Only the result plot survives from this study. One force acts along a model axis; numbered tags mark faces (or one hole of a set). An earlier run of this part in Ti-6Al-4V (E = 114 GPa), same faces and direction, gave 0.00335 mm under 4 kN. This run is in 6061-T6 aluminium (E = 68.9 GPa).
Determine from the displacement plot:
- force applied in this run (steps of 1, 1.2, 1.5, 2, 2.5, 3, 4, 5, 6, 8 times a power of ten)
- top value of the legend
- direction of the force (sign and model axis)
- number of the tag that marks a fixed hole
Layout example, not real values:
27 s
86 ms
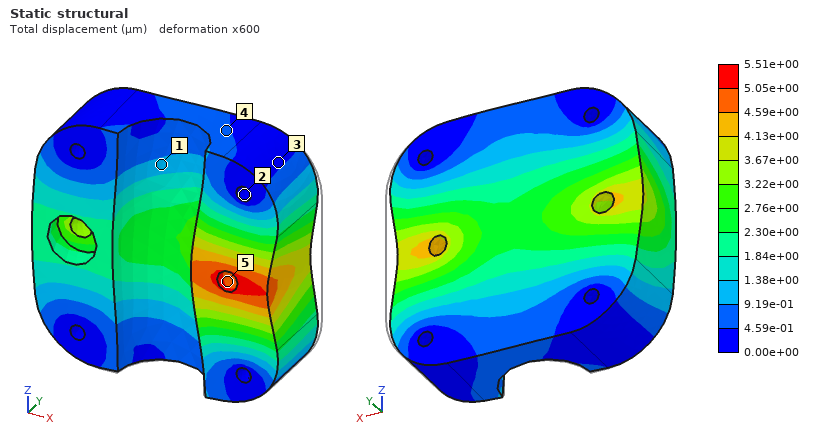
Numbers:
4 kN
5.51e+00 µm
-X
2
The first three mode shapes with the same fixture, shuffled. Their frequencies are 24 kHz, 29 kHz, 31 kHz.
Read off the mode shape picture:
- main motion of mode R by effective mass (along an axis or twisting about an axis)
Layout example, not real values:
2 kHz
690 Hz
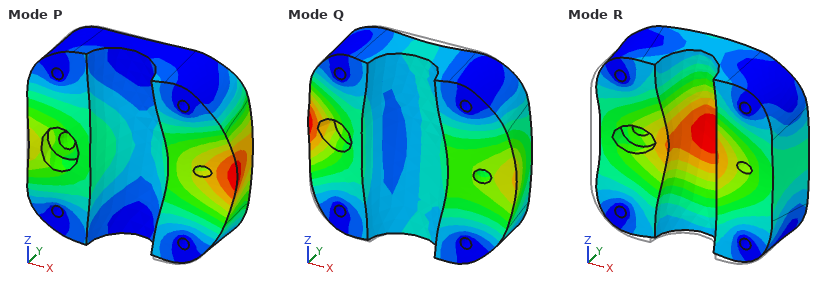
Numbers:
along Y
